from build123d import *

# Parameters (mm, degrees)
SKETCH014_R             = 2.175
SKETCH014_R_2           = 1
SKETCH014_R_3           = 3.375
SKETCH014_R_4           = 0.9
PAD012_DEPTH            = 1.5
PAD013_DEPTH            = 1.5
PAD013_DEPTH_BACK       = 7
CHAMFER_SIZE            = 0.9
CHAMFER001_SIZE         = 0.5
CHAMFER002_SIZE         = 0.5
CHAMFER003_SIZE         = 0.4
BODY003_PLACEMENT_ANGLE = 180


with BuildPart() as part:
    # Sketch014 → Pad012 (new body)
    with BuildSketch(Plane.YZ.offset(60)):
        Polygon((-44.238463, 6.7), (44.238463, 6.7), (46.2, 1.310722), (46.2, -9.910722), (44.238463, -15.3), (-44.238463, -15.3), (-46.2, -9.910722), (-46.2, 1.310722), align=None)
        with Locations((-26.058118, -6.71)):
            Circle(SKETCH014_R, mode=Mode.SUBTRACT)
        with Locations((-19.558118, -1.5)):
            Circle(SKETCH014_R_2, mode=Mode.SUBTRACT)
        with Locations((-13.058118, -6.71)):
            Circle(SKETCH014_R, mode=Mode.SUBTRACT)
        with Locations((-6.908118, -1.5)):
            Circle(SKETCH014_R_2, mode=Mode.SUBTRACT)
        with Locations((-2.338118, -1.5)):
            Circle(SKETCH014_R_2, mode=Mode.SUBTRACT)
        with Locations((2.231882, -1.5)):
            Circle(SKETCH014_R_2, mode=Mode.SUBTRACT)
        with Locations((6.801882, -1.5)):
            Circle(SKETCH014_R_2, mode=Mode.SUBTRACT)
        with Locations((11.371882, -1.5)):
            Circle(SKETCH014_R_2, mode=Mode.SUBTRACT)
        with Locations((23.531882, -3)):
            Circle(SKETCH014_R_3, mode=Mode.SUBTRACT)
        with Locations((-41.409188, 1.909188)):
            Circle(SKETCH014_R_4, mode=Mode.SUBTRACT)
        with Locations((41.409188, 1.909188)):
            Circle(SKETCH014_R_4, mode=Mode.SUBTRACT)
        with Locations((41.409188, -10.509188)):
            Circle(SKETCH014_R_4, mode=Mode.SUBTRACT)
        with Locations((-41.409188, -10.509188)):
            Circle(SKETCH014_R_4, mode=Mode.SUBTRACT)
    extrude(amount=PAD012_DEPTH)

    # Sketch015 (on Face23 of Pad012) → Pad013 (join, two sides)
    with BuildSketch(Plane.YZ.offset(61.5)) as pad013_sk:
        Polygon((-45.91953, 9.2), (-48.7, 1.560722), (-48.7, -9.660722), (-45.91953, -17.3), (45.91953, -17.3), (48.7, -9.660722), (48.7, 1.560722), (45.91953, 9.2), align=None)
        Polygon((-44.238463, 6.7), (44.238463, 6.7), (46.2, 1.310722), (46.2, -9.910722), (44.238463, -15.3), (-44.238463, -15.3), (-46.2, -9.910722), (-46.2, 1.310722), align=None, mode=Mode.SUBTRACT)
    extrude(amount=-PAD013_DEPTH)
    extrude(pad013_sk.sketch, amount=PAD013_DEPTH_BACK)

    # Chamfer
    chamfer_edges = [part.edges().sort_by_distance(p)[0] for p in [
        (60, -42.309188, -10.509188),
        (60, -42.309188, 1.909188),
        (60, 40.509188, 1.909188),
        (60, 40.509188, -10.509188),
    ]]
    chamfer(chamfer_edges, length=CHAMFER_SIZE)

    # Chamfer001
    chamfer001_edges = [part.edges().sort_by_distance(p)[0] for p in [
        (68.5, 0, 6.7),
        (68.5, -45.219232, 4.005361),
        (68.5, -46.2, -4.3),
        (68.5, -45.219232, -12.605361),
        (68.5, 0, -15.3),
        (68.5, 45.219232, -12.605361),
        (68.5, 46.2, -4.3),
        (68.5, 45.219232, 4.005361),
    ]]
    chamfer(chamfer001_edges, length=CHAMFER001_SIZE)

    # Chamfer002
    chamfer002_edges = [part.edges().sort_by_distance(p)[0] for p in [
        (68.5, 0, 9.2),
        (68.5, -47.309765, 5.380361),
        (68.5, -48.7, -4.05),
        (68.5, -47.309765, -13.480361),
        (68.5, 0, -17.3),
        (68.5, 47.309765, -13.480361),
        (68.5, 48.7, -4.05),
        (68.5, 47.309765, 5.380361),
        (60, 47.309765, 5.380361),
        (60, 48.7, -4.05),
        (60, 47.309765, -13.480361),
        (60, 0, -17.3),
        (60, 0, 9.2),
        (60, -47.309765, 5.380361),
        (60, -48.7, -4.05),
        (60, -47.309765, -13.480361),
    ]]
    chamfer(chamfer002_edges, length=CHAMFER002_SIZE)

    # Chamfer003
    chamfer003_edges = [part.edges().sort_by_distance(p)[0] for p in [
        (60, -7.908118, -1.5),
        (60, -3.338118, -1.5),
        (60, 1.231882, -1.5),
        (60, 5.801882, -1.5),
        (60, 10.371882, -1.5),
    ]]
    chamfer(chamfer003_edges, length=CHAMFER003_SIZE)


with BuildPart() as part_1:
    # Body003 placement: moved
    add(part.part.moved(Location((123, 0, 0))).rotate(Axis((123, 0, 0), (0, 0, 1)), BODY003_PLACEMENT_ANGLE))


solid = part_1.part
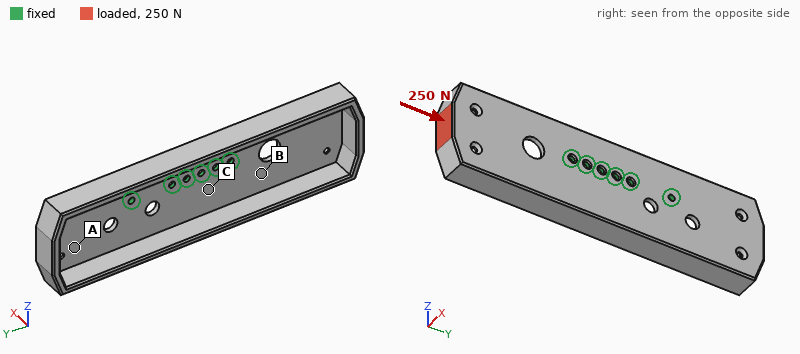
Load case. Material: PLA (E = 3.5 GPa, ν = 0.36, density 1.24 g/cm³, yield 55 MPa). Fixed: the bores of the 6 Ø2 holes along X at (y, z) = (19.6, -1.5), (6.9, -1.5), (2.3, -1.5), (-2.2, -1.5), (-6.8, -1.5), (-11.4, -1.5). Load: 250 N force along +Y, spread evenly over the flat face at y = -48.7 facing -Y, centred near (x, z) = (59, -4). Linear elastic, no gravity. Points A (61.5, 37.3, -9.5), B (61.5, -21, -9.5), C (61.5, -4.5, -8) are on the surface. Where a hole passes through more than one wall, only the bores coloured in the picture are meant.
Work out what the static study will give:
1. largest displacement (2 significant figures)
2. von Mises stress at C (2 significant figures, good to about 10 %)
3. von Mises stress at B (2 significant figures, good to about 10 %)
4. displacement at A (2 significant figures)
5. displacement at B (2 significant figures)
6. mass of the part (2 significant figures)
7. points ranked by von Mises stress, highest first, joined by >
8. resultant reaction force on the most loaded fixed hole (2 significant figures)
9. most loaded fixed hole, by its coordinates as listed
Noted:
1.0 mm
7.5 MPa
5.3 MPa
0.27 mm
0.21 mm
9.0 g
C > B > A
77 N
(-11.4, -1.5)
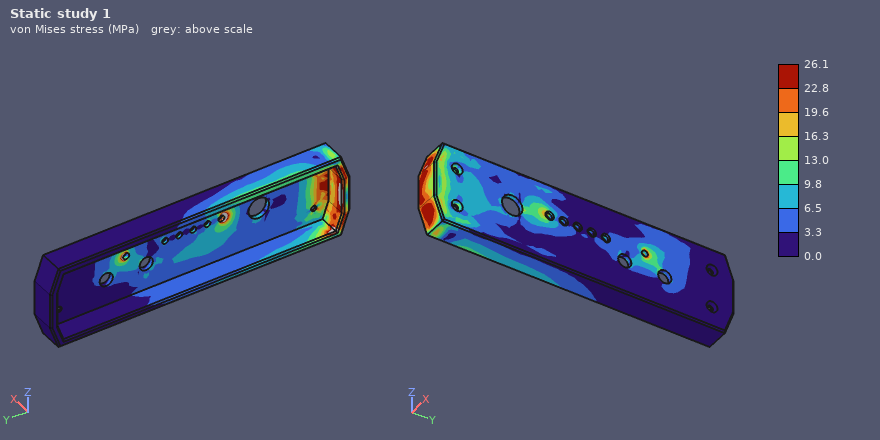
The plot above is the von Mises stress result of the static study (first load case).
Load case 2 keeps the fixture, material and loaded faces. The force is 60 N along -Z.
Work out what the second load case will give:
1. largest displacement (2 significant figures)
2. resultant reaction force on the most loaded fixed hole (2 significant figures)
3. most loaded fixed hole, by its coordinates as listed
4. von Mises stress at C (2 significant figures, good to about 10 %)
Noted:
1.1 mm
140 N
(-11.4, -1.5)
6.2 MPa
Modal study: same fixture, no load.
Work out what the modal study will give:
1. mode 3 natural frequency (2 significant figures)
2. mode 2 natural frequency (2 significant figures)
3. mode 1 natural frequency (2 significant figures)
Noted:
760 Hz
630 Hz
500 Hz
